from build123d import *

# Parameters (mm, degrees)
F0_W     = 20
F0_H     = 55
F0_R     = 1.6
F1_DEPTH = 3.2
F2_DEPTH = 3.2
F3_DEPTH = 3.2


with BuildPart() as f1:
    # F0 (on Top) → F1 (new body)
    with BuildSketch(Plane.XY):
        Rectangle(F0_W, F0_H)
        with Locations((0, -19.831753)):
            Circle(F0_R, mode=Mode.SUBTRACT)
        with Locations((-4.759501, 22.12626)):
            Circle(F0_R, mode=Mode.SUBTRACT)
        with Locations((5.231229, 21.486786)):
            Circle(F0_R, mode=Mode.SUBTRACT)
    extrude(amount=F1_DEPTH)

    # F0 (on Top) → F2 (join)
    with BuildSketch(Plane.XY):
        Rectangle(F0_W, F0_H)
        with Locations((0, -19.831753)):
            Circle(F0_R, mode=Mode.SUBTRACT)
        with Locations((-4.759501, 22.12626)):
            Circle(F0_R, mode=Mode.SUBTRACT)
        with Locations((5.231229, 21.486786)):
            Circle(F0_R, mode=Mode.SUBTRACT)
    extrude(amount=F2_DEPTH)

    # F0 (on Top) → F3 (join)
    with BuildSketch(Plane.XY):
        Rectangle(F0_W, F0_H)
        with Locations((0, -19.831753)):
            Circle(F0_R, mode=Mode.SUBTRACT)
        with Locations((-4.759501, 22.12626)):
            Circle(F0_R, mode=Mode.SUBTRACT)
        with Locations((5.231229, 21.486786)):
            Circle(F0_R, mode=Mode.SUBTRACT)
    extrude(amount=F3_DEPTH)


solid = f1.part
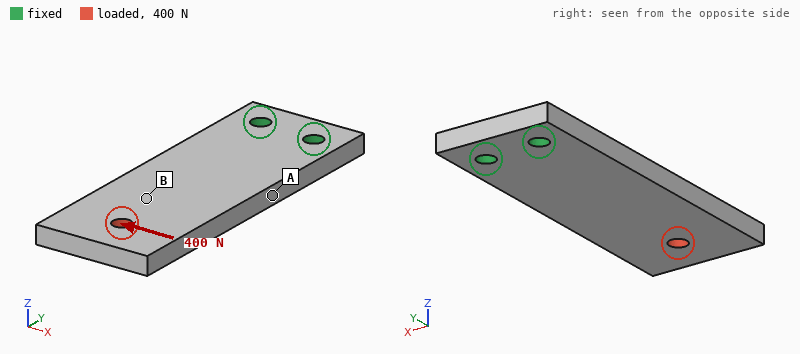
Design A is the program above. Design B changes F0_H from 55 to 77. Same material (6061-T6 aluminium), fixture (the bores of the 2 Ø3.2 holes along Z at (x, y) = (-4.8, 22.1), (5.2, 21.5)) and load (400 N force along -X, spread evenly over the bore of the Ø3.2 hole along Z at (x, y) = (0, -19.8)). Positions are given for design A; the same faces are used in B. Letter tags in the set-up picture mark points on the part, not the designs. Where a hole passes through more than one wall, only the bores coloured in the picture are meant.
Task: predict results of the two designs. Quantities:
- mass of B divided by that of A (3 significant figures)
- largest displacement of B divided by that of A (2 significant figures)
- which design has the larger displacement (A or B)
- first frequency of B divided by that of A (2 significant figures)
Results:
1.41
1.2
B
0.66
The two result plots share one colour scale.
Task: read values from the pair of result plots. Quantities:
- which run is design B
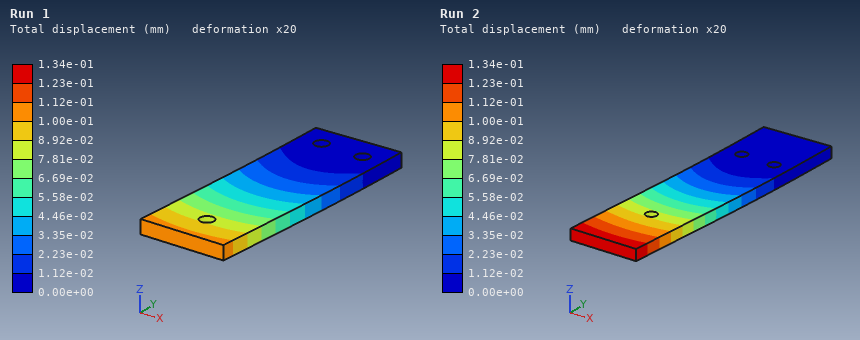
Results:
Run 2
